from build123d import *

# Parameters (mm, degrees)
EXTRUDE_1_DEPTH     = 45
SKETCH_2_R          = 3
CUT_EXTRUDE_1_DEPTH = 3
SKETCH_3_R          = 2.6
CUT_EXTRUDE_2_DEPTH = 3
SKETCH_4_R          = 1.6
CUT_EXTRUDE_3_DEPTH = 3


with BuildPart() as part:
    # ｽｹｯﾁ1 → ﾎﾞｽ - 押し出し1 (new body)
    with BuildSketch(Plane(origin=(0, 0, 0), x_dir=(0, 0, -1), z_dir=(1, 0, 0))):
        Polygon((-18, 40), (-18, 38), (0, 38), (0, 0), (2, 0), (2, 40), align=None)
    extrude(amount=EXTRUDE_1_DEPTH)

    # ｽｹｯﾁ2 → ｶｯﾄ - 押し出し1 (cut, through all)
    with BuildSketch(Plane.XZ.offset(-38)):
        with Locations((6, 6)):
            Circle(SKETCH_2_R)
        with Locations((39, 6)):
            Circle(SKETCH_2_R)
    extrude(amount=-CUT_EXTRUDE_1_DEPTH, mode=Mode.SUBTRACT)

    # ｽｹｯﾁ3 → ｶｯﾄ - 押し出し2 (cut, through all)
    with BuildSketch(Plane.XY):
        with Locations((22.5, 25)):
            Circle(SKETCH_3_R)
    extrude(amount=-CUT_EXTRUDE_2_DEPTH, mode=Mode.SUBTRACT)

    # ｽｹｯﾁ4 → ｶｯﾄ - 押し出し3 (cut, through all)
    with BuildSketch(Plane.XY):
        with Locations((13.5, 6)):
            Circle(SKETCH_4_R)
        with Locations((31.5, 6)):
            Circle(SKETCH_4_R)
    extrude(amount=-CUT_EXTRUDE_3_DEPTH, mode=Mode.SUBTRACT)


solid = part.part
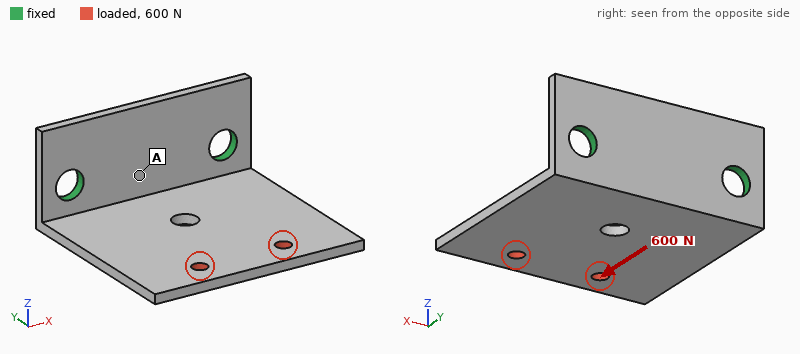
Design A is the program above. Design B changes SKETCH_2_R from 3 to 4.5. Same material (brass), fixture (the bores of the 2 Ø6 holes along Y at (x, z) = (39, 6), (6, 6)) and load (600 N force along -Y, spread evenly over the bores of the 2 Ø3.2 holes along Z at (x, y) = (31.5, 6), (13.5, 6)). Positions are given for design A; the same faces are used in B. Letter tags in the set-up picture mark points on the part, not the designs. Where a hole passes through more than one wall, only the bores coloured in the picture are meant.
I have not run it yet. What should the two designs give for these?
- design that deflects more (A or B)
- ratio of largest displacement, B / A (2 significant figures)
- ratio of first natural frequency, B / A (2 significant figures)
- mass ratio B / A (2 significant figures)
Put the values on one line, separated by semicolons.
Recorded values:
A; 0.47; 1.1; 0.97
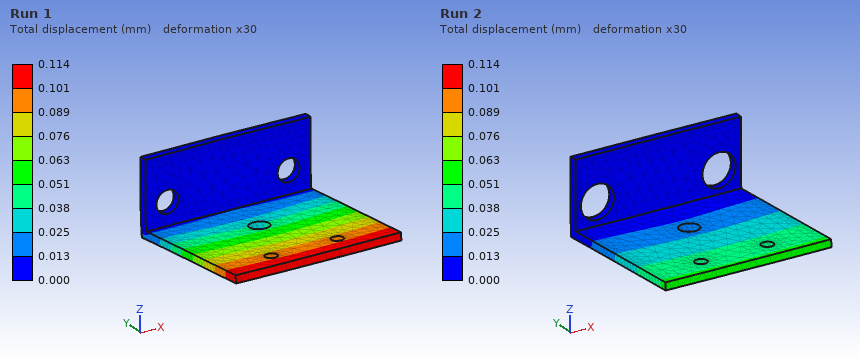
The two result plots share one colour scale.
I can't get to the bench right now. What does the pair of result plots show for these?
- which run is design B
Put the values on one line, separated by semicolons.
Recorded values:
Run 2
